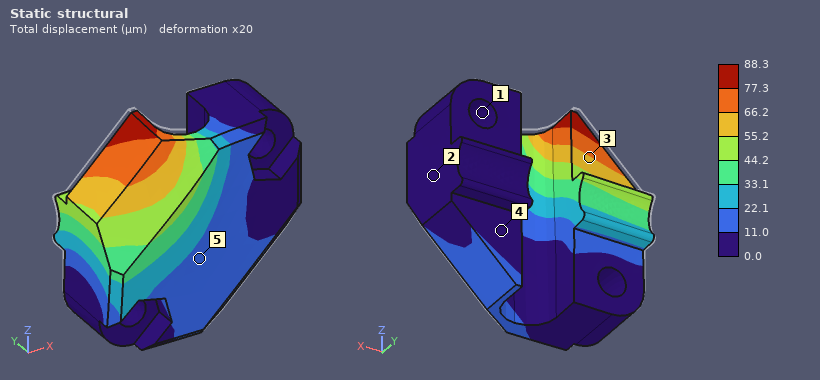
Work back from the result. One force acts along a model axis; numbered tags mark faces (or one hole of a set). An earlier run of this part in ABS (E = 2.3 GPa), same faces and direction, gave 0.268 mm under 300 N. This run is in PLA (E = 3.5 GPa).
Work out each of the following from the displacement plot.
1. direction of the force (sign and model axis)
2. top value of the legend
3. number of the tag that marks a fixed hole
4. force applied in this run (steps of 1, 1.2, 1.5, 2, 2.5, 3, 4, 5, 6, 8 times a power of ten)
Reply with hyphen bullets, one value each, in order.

- -Y
- 88.3 µm
- 1
- 150 N
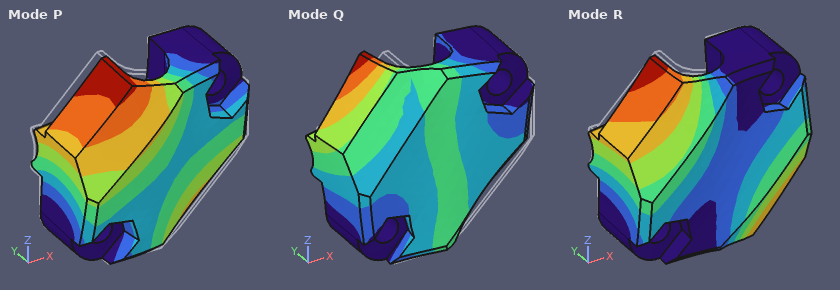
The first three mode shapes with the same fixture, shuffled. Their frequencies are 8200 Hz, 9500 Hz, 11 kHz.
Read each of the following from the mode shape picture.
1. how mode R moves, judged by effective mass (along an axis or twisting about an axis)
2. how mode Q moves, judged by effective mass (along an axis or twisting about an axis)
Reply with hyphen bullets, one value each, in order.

- along Y
- along X
